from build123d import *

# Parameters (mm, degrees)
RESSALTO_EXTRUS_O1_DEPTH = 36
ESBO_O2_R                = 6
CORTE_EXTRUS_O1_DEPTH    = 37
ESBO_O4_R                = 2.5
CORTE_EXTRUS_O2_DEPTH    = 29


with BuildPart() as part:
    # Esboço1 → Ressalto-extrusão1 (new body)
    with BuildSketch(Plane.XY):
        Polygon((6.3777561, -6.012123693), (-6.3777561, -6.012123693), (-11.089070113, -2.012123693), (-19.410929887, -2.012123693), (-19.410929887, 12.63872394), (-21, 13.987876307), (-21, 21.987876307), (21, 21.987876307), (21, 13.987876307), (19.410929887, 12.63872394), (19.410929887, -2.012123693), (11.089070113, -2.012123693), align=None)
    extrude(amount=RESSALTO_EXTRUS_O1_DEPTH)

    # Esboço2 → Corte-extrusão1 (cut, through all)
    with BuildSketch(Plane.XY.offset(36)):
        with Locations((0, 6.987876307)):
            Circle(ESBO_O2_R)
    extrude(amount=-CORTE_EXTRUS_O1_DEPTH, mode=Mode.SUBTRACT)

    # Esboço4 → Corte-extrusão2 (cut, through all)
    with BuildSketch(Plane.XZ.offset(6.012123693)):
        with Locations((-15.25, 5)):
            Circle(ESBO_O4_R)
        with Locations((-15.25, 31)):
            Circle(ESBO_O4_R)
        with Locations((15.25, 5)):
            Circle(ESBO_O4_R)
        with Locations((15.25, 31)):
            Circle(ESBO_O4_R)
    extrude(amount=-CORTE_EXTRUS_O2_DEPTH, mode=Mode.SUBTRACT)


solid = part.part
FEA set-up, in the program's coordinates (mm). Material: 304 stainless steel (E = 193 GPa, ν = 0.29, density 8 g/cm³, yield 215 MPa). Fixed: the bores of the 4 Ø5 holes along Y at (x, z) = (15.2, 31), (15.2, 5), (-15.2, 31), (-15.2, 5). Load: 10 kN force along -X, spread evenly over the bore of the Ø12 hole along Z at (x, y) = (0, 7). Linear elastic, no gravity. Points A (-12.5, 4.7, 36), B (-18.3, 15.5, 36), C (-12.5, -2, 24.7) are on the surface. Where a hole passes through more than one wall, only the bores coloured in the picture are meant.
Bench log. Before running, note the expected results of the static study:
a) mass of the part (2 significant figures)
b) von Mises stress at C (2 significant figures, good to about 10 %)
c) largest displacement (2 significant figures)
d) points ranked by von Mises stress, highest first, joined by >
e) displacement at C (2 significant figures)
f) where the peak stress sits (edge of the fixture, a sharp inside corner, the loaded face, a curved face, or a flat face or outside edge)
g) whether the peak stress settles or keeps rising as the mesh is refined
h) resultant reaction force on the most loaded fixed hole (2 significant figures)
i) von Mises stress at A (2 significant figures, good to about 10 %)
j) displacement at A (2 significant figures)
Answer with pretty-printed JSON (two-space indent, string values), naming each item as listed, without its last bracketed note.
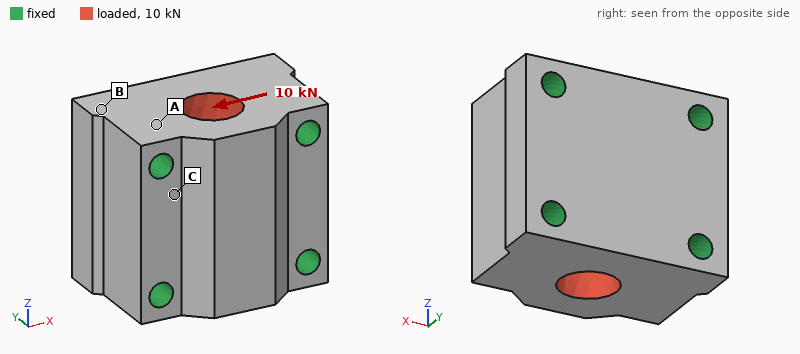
{
  "mass of the part": "250 g",
  "von Mises stress at C": "7.3 MPa",
  "largest displacement": "0.88 µm",
  "points ranked by von Mises stress, highest first, joined by >": "C > A > B",
  "displacement at C": "0.48 µm",
  "where the peak stress sits": "edge of the fixture",
  "whether the peak stress settles or keeps rising as the mesh is refined": "keeps rising",
  "resultant reaction force on the most loaded fixed hole": "2.6 kN",
  "von Mises stress at A": "4.3 MPa",
  "displacement at A": "0.15 µm"
}
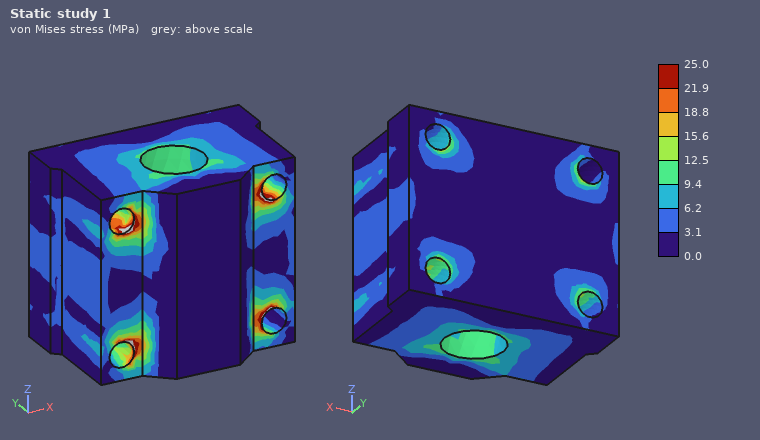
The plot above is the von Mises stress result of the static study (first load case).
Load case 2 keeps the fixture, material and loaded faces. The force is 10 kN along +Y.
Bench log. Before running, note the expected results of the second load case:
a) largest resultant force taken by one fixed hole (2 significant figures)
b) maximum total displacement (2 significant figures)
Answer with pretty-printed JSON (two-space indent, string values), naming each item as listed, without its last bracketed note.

{
  "largest resultant force taken by one fixed hole": "2.5 kN",
  "maximum total displacement": "1.6 µm"
}
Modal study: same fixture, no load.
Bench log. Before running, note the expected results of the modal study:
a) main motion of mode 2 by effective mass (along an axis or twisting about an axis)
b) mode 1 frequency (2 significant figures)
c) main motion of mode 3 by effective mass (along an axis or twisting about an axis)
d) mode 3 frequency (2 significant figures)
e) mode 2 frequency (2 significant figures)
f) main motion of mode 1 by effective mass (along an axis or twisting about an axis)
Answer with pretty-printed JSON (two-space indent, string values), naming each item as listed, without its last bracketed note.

{
  "main motion of mode 2 by effective mass": "along Z",
  "mode 1 frequency": "42 kHz",
  "main motion of mode 3 by effective mass": "along Z",
  "mode 3 frequency": "50 kHz",
  "mode 2 frequency": "44 kHz",
  "main motion of mode 1 by effective mass": "along Y"
}
